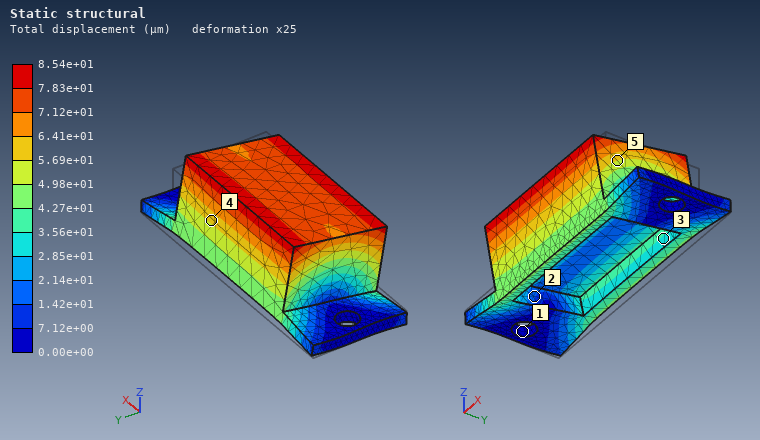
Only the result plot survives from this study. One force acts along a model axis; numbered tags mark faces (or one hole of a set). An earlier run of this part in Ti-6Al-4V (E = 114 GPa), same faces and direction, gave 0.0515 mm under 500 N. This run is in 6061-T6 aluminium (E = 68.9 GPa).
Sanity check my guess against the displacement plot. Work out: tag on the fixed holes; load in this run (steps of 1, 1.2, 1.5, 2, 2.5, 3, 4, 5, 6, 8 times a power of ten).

1
500 N
